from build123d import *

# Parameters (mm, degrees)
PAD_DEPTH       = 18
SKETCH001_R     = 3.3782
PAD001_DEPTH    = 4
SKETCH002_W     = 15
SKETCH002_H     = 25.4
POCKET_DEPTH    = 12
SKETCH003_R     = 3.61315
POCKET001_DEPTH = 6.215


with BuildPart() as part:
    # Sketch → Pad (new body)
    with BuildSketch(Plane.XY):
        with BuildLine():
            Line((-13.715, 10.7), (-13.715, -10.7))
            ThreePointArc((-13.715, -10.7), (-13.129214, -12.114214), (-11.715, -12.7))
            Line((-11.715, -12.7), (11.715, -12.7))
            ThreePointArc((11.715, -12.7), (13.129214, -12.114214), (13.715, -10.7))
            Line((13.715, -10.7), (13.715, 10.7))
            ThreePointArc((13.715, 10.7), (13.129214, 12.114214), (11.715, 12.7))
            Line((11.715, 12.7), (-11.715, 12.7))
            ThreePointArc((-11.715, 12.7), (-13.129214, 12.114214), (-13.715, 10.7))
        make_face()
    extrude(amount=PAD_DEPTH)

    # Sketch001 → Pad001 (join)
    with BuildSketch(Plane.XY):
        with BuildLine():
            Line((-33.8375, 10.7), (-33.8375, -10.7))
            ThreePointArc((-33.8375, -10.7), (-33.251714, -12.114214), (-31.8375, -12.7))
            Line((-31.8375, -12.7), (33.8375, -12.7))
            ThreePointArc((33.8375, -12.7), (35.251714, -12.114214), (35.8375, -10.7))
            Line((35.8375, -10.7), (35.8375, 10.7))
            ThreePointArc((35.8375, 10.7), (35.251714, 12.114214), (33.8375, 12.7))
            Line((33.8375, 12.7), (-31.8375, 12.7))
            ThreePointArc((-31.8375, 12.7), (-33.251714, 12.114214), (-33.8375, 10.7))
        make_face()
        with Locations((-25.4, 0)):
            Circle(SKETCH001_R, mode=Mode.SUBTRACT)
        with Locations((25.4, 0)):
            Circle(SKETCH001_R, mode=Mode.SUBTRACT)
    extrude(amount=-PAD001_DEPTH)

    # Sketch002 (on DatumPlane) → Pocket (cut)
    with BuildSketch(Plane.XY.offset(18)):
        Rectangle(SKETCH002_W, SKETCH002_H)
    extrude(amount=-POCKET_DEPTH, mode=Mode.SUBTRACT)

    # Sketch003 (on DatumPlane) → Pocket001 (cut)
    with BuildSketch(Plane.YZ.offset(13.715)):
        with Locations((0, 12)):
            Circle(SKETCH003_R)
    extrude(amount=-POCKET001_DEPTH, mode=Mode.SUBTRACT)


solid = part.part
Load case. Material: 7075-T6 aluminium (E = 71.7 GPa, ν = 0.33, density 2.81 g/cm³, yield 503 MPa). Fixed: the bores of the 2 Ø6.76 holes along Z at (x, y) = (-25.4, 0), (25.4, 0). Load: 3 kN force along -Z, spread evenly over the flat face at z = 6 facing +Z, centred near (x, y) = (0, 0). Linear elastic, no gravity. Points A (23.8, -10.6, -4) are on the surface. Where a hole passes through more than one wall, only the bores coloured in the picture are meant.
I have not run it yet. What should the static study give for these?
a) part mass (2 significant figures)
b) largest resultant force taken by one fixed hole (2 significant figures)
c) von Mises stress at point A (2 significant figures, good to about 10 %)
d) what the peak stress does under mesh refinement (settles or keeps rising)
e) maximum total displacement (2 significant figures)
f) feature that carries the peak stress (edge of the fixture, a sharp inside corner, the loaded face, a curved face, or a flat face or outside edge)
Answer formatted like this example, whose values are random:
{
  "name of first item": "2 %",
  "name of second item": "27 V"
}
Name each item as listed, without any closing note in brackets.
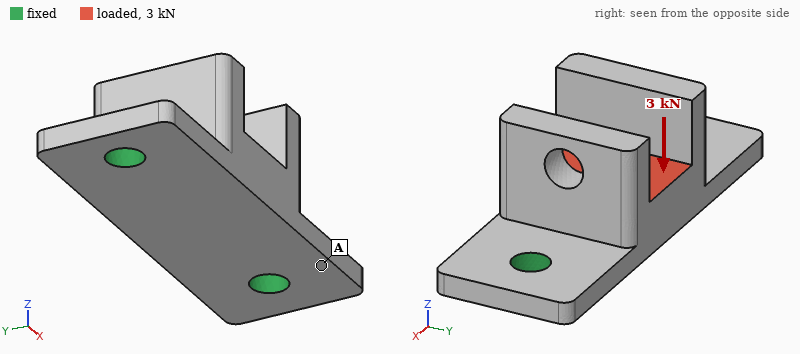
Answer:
{
  "part mass": "41 g",
  "largest resultant force taken by one fixed hole": "1.9 kN",
  "von Mises stress at point A": "39 MPa",
  "what the peak stress does under mesh refinement": "keeps rising",
  "maximum total displacement": "49 µm",
  "feature that carries the peak stress": "edge of the fixture"
}
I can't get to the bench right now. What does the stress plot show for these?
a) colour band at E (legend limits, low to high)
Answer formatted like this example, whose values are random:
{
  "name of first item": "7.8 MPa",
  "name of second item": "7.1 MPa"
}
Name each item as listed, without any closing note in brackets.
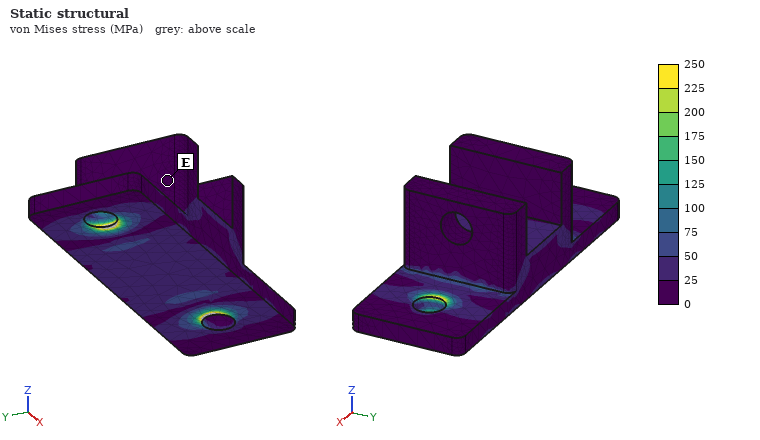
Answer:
{
  "colour band at E": "0 to 25 MPa"
}
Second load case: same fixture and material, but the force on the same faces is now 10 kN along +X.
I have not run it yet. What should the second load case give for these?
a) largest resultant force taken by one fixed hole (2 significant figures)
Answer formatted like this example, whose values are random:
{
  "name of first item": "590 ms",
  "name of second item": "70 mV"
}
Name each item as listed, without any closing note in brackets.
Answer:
{
  "largest resultant force taken by one fixed hole": "5.5 kN"
}
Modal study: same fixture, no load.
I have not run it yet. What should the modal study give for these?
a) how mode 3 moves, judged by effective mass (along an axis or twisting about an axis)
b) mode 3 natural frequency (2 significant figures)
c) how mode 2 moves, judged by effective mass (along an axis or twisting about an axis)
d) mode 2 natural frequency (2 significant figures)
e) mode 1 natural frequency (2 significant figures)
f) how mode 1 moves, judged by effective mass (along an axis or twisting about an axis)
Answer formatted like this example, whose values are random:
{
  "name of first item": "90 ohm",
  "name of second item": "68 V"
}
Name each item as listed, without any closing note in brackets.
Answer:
{
  "how mode 3 moves, judged by effective mass": "along X",
  "mode 3 natural frequency": "11 kHz",
  "how mode 2 moves, judged by effective mass": "along Z",
  "mode 2 natural frequency": "7800 Hz",
  "mode 1 natural frequency": "4600 Hz",
  "how mode 1 moves, judged by effective mass": "along Y"
}
